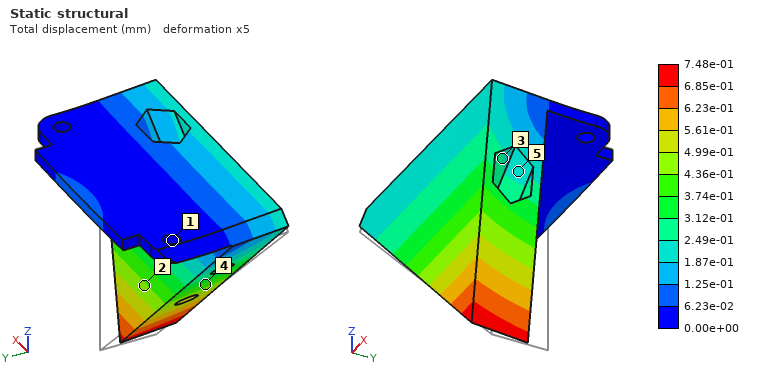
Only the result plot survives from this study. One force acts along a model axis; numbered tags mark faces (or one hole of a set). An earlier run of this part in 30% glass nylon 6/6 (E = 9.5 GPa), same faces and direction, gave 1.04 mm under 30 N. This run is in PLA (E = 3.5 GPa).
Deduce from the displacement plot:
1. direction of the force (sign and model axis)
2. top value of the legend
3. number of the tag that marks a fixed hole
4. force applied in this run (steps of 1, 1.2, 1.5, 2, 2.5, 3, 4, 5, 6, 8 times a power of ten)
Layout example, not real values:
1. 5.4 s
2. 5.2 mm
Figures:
1. -Y
2. 7.48e-01 mm
3. 1
4. 8 N
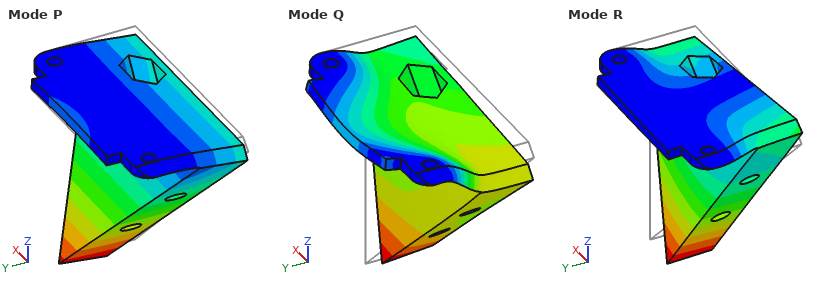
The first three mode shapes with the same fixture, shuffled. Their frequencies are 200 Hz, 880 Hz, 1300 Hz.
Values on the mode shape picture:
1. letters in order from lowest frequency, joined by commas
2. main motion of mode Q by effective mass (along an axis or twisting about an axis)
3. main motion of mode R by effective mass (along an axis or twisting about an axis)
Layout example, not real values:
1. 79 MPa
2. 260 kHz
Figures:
1. P, R, Q
2. along Z
3. along X
